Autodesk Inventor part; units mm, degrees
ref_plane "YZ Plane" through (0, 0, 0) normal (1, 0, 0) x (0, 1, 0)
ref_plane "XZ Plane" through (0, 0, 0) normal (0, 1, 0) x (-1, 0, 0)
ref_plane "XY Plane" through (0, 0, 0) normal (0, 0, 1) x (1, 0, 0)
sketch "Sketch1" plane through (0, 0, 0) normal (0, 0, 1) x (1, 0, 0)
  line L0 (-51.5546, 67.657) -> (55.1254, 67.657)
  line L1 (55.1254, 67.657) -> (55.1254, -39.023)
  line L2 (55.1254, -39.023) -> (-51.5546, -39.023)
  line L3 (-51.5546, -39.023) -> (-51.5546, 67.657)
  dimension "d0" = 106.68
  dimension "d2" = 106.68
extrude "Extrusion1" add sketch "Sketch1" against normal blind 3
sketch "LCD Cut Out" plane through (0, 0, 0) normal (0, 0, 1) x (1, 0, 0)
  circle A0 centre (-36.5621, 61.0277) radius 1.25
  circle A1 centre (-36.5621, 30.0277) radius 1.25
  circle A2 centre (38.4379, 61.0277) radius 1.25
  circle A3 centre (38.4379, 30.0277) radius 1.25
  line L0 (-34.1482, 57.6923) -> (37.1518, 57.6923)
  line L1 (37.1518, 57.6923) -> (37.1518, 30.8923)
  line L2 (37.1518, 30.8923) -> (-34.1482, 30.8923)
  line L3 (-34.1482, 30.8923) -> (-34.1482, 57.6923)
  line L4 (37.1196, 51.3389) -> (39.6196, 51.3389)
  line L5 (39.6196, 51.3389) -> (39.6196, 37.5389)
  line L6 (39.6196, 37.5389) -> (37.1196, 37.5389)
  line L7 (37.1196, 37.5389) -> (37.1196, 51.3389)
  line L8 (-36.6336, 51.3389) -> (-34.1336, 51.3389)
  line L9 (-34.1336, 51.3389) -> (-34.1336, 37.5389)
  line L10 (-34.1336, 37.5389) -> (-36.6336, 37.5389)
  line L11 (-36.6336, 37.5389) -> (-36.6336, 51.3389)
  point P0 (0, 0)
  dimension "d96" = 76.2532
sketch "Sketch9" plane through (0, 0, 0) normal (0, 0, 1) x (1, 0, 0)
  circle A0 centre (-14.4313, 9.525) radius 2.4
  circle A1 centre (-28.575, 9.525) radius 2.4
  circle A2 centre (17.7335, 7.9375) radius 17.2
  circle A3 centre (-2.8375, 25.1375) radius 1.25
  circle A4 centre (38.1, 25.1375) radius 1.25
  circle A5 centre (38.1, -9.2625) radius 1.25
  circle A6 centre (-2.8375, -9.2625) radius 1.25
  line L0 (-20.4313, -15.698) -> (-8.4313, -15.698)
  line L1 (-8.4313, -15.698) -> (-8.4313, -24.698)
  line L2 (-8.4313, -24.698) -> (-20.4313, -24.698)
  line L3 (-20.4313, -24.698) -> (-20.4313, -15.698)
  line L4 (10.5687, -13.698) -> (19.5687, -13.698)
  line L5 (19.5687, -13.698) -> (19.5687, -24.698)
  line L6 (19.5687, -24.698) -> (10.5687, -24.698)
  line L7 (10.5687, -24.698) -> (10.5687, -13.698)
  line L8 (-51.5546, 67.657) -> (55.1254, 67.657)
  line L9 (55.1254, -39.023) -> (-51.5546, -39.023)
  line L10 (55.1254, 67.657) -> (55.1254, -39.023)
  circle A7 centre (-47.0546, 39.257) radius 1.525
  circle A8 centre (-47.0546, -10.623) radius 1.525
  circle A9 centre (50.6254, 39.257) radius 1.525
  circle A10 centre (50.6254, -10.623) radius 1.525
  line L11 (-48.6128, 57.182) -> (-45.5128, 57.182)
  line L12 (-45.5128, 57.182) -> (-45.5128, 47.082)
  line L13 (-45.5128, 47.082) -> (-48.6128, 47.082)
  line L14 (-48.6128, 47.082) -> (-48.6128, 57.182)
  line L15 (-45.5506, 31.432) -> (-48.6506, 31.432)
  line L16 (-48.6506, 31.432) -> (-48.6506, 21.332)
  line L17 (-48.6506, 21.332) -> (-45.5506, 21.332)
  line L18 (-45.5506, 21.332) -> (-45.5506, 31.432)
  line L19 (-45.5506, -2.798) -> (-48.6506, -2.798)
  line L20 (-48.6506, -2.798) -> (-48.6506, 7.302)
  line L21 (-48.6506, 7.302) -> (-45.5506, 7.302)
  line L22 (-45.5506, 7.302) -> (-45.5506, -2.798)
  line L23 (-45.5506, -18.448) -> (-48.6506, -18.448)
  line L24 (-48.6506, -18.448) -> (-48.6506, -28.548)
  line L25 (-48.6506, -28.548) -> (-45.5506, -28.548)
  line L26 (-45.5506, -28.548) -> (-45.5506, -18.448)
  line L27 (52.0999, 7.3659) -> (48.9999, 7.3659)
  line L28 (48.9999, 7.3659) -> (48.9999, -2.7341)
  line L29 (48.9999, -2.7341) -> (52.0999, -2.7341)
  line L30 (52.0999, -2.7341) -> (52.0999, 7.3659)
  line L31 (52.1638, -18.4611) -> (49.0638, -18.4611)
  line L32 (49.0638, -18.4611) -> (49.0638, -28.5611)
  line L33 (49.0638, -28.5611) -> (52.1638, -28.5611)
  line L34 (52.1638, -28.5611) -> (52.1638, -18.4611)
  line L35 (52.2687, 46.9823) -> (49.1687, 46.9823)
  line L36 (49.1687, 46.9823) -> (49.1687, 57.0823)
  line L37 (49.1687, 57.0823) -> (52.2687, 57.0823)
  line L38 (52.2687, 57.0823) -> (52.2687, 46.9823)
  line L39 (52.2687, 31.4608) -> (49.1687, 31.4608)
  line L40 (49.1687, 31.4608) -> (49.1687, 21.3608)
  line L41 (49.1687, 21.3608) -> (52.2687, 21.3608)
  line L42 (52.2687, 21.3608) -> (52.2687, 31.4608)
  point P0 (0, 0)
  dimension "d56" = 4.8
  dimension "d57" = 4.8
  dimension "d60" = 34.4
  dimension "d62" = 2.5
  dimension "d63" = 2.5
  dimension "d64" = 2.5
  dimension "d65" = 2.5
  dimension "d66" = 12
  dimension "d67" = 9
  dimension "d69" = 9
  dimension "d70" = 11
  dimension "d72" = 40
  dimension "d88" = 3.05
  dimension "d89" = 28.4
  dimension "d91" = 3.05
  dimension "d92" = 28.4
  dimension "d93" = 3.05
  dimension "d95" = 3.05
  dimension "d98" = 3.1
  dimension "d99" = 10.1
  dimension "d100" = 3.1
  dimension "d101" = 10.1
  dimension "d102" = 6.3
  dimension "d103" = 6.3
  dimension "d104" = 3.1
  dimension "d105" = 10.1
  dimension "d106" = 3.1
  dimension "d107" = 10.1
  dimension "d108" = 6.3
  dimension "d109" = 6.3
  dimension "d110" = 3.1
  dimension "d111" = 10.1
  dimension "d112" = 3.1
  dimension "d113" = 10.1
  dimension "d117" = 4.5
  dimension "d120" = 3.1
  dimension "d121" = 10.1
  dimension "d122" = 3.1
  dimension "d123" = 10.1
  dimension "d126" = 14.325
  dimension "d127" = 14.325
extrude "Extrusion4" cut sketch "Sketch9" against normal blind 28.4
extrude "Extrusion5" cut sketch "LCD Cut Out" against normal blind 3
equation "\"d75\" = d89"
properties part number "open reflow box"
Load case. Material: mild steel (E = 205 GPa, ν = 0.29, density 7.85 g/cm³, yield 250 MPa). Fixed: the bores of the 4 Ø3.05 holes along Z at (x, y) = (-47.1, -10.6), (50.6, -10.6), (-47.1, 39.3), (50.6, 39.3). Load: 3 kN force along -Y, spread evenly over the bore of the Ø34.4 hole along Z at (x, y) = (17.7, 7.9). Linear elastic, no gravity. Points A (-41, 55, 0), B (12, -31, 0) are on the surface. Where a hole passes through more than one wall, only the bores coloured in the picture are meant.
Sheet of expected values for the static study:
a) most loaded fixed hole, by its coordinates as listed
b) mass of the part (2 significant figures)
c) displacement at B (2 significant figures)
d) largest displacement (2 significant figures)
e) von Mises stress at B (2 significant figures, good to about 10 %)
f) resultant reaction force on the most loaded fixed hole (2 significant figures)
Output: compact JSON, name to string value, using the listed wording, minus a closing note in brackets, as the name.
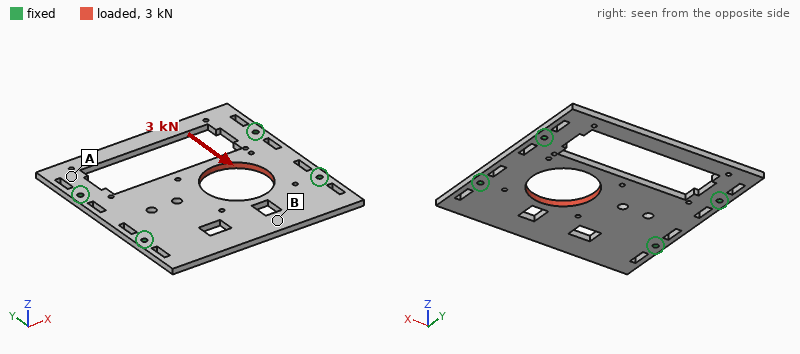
{"most loaded fixed hole, by its coordinates as listed": "(50.6, -10.6)", "mass of the part": "190 g", "displacement at B": "6.4 µm", "largest displacement": "13 µm", "von Mises stress at B": "18 MPa", "resultant reaction force on the most loaded fixed hole": "1.2 kN"}
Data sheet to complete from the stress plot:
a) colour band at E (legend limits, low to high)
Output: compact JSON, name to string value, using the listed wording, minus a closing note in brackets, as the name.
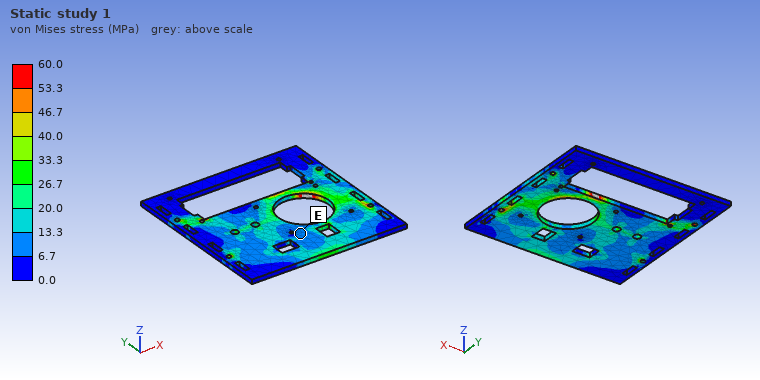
{"colour band at E": "6.7 to 13.3 MPa"}
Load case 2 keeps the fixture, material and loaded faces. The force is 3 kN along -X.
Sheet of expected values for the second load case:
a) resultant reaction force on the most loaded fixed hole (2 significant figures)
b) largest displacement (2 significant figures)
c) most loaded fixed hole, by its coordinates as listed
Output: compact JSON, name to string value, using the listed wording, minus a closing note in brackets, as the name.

{"resultant reaction force on the most loaded fixed hole": "1.3 kN", "largest displacement": "5.8 µm", "most loaded fixed hole, by its coordinates as listed": "(50.6, -10.6)"}
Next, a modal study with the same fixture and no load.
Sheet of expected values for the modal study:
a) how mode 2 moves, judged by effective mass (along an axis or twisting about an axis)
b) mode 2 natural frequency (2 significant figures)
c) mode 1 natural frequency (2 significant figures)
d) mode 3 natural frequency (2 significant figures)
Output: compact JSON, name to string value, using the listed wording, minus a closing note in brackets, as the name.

{"how mode 2 moves, judged by effective mass": "along Z", "mode 2 natural frequency": "1200 Hz", "mode 1 natural frequency": "1100 Hz", "mode 3 natural frequency": "1700 Hz"}
